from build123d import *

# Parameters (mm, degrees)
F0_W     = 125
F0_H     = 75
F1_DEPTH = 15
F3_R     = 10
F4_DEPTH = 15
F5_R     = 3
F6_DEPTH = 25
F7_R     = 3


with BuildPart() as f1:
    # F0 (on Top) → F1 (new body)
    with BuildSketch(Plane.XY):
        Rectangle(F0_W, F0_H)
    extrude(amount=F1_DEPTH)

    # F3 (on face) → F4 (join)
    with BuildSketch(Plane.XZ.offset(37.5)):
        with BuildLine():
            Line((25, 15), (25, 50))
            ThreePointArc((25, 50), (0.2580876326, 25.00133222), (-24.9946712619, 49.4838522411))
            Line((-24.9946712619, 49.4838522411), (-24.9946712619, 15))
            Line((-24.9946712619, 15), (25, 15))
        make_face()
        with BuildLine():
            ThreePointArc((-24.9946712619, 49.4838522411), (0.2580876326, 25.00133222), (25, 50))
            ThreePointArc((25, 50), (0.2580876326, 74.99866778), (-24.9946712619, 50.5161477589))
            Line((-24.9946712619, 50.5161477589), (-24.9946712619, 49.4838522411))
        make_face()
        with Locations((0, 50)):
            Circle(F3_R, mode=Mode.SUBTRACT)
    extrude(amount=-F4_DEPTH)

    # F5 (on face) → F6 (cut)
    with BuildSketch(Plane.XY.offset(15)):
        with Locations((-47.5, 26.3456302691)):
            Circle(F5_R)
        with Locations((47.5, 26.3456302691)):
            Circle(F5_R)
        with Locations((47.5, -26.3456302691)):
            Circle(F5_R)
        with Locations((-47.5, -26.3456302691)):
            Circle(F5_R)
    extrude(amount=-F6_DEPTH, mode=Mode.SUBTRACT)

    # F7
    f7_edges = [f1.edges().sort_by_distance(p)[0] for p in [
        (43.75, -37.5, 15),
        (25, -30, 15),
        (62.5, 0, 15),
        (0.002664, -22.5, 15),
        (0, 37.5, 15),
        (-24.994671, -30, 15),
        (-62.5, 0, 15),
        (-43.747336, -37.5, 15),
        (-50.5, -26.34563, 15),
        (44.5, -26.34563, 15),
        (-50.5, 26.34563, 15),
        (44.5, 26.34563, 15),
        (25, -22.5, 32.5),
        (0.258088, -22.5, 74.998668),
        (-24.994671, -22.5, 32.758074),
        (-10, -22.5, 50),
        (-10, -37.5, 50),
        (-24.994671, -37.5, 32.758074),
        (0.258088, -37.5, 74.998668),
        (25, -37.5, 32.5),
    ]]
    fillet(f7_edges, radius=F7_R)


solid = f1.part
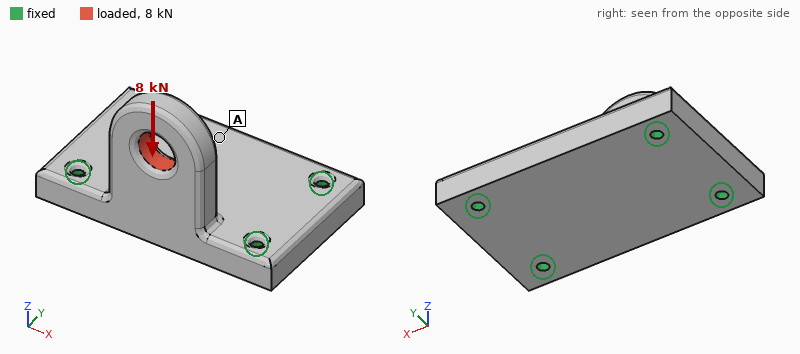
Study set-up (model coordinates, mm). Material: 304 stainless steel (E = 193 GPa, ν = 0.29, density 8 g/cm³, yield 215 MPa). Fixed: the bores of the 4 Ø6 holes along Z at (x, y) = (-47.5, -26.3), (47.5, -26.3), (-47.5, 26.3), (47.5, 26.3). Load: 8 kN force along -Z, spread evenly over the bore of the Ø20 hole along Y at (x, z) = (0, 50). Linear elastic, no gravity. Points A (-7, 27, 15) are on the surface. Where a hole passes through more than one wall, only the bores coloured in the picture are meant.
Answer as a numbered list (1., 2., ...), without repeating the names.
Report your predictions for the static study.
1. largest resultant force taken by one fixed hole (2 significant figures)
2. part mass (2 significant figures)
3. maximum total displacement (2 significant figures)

1. 4.4 kN
2. 1.4 kg
3. 30 µm
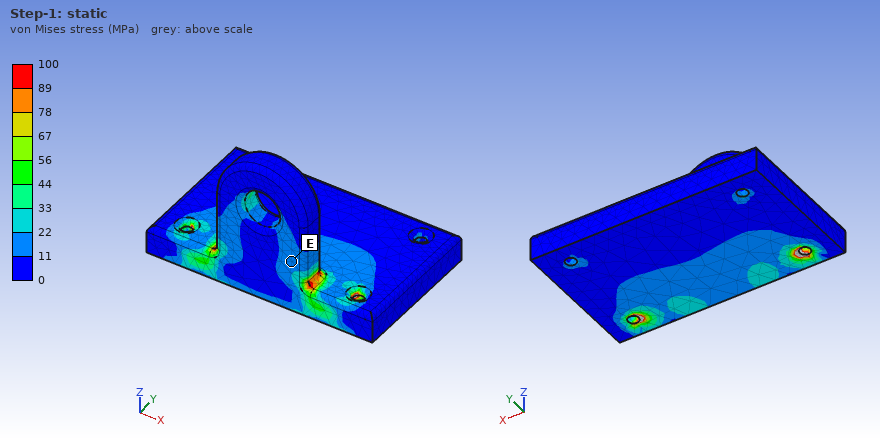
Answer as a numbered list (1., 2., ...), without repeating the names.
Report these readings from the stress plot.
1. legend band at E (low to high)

1. 11 to 22 MPa
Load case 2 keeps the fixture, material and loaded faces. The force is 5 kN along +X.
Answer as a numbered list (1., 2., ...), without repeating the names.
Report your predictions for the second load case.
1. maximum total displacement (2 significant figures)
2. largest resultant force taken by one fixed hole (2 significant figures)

1. 27 µm
2. 3.4 kN
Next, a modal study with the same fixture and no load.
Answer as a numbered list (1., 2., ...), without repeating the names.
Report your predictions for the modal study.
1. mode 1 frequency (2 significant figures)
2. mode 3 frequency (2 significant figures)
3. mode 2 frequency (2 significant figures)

1. 2500 Hz
2. 5400 Hz
3. 5300 Hz
